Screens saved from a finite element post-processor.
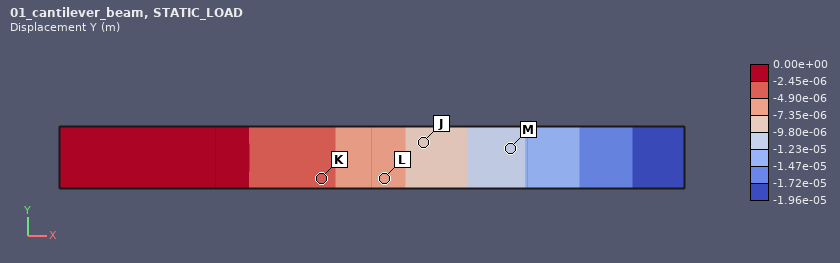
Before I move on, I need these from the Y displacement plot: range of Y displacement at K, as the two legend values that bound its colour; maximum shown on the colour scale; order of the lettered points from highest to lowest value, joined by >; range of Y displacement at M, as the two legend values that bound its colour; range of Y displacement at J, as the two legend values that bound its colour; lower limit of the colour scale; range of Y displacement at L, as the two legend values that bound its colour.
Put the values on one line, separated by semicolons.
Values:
-4.90e-06 to -2.45e-06 m; 0.00e+00 m; K > L > J > M; -1.23e-05 to -9.80e-06 m; -9.80e-06 to -7.35e-06 m; -1.96e-05 m; -7.35e-06 to -4.90e-06 m
